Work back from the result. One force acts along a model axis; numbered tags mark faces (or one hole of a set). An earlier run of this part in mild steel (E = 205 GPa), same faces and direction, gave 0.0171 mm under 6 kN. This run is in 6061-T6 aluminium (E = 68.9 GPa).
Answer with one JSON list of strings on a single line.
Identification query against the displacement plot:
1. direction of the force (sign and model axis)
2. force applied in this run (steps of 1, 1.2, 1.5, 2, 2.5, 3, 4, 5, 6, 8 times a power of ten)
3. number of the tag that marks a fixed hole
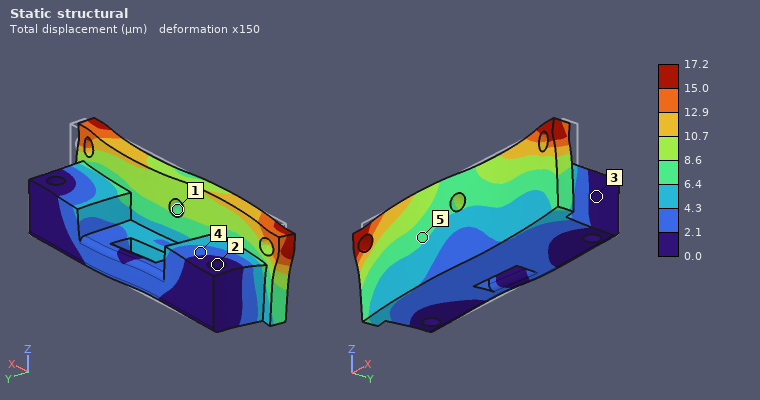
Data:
["-X", "2 kN", "2"]
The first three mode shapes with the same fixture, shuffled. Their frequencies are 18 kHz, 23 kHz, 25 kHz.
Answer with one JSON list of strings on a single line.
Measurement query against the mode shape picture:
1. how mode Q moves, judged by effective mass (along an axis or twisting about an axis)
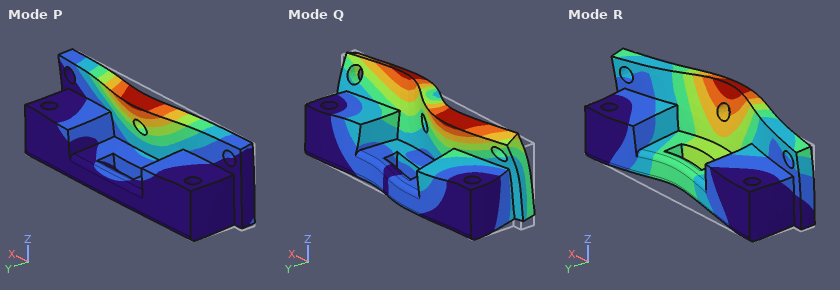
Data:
["along X"]
